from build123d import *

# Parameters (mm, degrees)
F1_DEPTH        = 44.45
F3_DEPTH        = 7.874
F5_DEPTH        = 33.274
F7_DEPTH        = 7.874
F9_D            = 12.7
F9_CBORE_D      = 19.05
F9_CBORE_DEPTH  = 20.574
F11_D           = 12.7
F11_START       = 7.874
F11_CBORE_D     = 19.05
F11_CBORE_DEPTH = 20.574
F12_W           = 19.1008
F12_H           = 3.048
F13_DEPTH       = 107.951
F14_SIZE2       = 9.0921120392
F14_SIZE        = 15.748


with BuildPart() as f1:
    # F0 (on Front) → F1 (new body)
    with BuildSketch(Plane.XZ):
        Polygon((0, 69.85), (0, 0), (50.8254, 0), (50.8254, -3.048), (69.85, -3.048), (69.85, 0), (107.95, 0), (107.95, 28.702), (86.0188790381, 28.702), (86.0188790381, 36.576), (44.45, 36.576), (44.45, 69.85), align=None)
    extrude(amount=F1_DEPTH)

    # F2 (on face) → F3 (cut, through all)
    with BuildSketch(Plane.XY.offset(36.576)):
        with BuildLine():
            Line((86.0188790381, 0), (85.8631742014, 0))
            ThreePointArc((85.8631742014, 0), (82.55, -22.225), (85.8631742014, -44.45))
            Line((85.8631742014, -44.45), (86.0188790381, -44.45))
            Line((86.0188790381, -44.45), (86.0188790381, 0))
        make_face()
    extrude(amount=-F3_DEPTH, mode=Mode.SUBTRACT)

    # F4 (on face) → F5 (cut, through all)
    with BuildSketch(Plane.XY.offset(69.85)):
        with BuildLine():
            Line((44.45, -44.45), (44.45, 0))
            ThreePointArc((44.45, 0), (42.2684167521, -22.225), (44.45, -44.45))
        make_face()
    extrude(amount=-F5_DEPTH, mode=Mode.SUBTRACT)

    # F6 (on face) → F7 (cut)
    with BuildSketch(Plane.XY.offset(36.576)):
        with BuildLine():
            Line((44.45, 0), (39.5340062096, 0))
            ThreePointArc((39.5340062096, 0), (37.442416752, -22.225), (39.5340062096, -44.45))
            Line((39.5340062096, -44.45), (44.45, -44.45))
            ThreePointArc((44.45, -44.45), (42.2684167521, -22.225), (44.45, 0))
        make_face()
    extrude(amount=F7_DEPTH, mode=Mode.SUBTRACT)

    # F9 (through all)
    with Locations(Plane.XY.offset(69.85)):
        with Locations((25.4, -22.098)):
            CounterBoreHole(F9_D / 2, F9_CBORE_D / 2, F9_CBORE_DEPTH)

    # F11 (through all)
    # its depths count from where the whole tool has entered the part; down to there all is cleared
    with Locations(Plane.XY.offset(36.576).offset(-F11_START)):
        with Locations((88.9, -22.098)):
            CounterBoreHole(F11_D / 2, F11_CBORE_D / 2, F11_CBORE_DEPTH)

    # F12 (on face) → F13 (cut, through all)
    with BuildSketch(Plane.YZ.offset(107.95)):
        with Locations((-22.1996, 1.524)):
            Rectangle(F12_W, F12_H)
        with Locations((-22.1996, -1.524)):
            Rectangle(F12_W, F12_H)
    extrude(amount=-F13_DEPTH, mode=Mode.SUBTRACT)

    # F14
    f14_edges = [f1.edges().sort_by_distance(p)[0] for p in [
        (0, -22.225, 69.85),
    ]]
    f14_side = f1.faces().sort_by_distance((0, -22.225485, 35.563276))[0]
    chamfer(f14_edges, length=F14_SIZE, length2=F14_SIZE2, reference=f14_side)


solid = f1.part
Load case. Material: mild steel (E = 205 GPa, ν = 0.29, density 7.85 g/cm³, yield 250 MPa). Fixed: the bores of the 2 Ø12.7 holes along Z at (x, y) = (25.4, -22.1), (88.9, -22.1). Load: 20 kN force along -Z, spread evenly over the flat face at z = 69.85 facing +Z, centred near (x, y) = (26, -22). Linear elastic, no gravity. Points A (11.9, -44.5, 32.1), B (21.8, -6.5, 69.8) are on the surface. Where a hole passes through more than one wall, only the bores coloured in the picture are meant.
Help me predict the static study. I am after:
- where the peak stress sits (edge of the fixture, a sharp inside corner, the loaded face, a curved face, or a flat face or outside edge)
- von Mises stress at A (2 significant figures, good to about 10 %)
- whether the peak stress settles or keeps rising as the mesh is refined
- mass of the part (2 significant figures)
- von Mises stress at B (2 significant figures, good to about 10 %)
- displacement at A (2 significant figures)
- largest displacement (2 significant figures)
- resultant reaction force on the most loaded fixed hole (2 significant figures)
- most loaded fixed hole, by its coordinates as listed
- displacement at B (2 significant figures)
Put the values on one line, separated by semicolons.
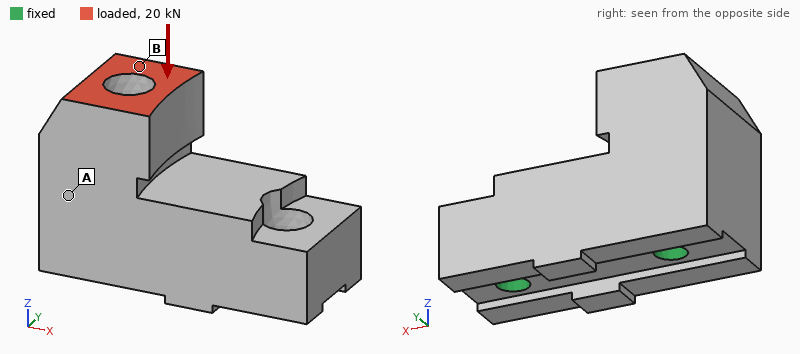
edge of the fixture; 4.9 MPa; keeps rising; 1.6 kg; 16 MPa; 0.99 µm; 5.4 µm; 20 kN; (25.4, -22.1); 3.7 µm
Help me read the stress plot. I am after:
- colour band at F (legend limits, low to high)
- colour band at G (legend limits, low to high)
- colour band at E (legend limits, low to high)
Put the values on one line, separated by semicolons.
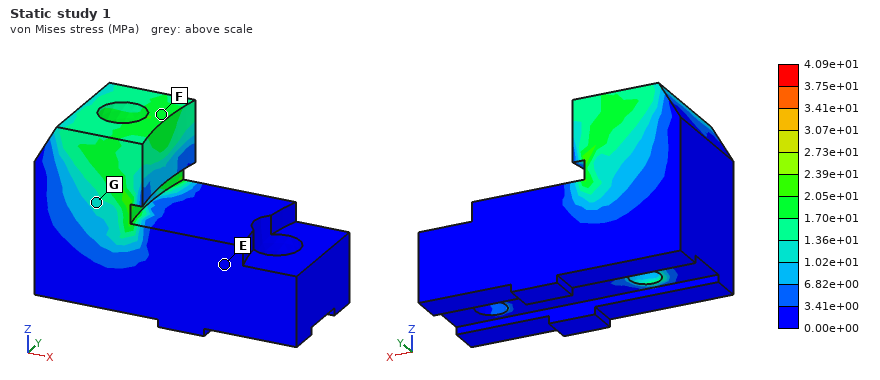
1.70e+01 to 2.05e+01 MPa; 1.02e+01 to 1.36e+01 MPa; 0.00e+00 to 3.41e+00 MPa
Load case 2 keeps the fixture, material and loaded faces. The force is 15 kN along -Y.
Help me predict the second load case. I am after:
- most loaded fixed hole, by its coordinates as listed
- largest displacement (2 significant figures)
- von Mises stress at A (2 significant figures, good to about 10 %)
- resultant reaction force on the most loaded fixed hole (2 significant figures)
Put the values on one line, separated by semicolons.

(25.4, -22.1); 17 µm; 20 MPa; 15 kN
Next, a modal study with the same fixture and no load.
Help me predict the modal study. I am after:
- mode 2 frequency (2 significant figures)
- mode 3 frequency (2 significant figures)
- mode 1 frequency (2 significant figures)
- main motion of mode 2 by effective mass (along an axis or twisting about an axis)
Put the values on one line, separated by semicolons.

13 kHz; 14 kHz; 8700 Hz; along Z
